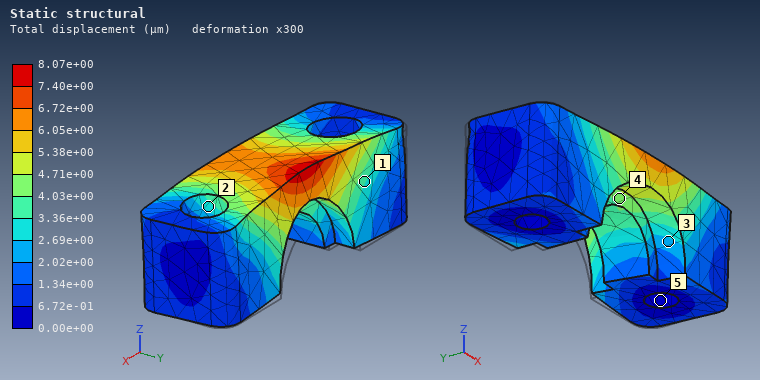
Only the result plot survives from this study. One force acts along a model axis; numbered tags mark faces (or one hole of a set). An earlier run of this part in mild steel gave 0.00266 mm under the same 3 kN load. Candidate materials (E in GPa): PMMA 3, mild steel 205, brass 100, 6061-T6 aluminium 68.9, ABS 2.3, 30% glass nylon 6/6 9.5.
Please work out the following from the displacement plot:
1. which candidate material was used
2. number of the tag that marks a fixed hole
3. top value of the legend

6061-T6 aluminium
5
8.07e+00 µm
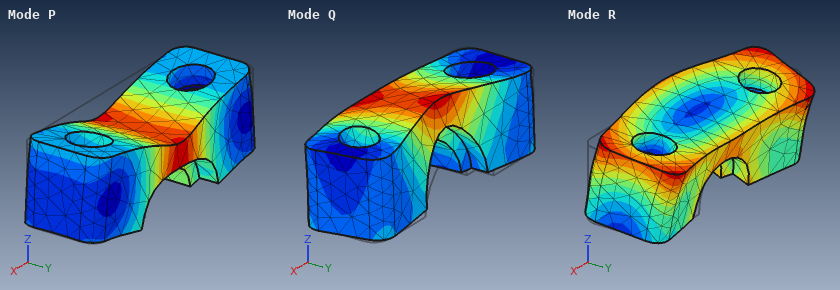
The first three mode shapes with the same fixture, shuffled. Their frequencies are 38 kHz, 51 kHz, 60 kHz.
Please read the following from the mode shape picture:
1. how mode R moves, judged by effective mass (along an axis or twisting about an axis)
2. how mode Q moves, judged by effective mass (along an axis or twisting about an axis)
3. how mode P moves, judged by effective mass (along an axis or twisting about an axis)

twisting about X
along Y
along Z
